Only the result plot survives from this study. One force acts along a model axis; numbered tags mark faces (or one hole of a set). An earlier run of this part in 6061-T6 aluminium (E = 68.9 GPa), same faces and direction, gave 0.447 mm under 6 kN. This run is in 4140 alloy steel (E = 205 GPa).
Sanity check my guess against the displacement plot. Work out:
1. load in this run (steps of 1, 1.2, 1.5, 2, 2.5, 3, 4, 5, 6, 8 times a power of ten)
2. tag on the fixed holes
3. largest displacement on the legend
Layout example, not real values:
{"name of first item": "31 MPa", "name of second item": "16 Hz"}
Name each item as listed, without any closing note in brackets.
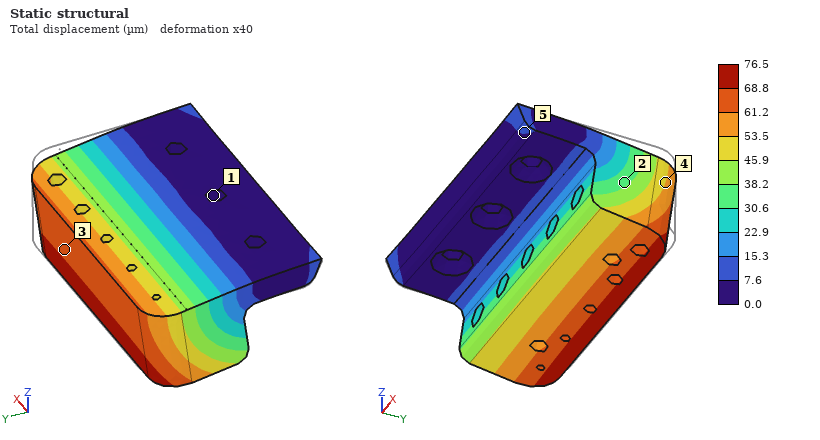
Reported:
{"load in this run": "3 kN", "tag on the fixed holes": "1", "largest displacement on the legend": "76.5 µm"}
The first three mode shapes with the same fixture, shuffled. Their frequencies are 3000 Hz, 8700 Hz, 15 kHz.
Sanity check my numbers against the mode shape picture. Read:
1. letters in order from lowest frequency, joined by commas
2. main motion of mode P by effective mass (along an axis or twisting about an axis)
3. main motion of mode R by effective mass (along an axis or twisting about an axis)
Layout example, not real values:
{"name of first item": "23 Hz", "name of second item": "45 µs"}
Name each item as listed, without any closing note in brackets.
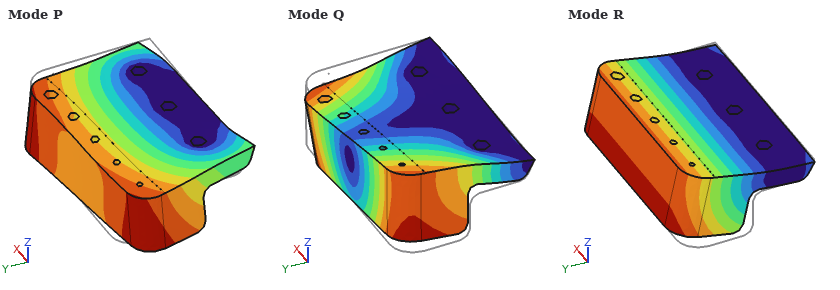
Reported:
{"letters in order from lowest frequency, joined by commas": "R, Q, P", "main motion of mode P by effective mass": "along X", "main motion of mode R by effective mass": "along Z"}
